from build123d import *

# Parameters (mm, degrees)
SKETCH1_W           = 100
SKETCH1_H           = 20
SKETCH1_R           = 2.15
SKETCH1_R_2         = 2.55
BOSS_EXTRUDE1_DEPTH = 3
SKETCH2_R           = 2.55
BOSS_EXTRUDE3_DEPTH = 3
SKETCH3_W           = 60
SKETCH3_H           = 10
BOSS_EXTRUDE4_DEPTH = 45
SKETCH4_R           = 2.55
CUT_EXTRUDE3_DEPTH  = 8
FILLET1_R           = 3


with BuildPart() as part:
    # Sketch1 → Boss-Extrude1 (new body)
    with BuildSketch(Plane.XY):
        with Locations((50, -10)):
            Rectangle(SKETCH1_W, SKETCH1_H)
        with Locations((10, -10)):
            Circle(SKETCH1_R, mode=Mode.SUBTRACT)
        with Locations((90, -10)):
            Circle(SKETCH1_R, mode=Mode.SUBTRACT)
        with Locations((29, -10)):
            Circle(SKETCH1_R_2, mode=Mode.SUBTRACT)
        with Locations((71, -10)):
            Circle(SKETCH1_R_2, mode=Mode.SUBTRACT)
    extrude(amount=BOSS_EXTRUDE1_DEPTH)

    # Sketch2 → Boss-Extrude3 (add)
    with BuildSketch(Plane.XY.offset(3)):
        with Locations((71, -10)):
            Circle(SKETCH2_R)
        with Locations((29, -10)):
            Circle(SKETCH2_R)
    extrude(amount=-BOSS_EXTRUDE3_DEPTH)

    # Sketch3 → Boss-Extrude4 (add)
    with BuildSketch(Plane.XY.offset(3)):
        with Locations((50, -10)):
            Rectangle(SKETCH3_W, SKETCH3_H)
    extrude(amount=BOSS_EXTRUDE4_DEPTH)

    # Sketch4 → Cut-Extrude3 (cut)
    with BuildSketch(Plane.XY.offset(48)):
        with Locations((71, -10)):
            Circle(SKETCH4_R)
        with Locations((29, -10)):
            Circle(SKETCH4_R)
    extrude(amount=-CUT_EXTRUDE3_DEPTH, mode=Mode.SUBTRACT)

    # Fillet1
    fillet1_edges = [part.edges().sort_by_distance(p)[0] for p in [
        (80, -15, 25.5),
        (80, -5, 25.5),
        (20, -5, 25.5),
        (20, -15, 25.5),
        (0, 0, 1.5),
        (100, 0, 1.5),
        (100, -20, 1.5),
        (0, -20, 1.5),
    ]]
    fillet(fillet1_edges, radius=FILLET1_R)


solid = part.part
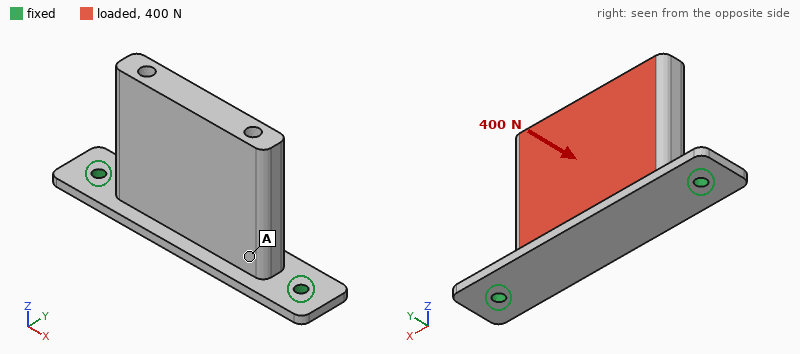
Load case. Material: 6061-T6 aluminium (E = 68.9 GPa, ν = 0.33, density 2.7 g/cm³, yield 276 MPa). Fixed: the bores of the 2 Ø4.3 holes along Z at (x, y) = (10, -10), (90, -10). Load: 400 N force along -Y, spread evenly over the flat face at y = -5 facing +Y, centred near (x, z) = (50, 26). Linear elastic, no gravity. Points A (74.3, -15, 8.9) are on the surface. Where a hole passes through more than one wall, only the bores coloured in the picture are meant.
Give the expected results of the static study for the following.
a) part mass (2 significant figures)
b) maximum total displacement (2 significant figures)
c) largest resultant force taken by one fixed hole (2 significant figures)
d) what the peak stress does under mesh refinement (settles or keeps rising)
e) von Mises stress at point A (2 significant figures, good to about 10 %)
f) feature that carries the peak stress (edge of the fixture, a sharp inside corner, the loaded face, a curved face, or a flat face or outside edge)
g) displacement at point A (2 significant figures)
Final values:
87 g
0.52 mm
200 N
keeps rising
16 MPa
edge of the fixture
0.100 mm
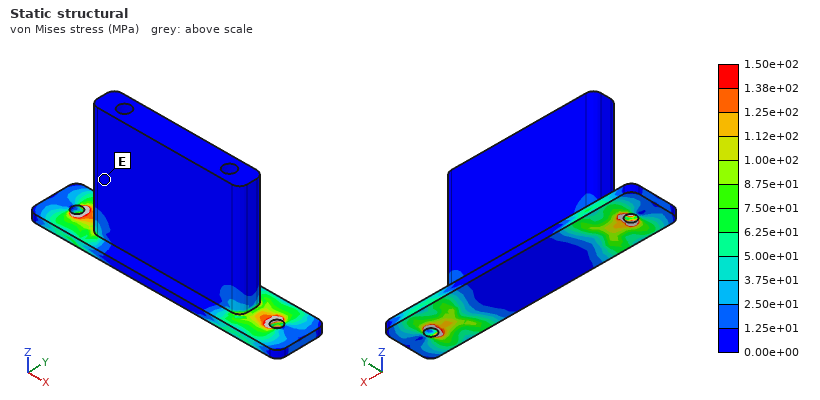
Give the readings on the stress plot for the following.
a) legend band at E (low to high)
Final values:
0.00e+00 to 1.25e+01 MPa
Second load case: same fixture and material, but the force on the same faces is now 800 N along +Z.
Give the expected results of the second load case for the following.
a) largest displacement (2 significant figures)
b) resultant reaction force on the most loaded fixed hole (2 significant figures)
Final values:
0.22 mm
460 N
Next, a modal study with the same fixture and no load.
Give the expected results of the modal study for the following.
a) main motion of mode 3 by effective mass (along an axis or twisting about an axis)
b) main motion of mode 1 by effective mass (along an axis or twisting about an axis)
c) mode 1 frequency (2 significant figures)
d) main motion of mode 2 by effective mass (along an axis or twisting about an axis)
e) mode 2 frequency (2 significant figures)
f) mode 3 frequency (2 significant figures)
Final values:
along X
along Y
640 Hz
along Z
3100 Hz
3500 Hz
